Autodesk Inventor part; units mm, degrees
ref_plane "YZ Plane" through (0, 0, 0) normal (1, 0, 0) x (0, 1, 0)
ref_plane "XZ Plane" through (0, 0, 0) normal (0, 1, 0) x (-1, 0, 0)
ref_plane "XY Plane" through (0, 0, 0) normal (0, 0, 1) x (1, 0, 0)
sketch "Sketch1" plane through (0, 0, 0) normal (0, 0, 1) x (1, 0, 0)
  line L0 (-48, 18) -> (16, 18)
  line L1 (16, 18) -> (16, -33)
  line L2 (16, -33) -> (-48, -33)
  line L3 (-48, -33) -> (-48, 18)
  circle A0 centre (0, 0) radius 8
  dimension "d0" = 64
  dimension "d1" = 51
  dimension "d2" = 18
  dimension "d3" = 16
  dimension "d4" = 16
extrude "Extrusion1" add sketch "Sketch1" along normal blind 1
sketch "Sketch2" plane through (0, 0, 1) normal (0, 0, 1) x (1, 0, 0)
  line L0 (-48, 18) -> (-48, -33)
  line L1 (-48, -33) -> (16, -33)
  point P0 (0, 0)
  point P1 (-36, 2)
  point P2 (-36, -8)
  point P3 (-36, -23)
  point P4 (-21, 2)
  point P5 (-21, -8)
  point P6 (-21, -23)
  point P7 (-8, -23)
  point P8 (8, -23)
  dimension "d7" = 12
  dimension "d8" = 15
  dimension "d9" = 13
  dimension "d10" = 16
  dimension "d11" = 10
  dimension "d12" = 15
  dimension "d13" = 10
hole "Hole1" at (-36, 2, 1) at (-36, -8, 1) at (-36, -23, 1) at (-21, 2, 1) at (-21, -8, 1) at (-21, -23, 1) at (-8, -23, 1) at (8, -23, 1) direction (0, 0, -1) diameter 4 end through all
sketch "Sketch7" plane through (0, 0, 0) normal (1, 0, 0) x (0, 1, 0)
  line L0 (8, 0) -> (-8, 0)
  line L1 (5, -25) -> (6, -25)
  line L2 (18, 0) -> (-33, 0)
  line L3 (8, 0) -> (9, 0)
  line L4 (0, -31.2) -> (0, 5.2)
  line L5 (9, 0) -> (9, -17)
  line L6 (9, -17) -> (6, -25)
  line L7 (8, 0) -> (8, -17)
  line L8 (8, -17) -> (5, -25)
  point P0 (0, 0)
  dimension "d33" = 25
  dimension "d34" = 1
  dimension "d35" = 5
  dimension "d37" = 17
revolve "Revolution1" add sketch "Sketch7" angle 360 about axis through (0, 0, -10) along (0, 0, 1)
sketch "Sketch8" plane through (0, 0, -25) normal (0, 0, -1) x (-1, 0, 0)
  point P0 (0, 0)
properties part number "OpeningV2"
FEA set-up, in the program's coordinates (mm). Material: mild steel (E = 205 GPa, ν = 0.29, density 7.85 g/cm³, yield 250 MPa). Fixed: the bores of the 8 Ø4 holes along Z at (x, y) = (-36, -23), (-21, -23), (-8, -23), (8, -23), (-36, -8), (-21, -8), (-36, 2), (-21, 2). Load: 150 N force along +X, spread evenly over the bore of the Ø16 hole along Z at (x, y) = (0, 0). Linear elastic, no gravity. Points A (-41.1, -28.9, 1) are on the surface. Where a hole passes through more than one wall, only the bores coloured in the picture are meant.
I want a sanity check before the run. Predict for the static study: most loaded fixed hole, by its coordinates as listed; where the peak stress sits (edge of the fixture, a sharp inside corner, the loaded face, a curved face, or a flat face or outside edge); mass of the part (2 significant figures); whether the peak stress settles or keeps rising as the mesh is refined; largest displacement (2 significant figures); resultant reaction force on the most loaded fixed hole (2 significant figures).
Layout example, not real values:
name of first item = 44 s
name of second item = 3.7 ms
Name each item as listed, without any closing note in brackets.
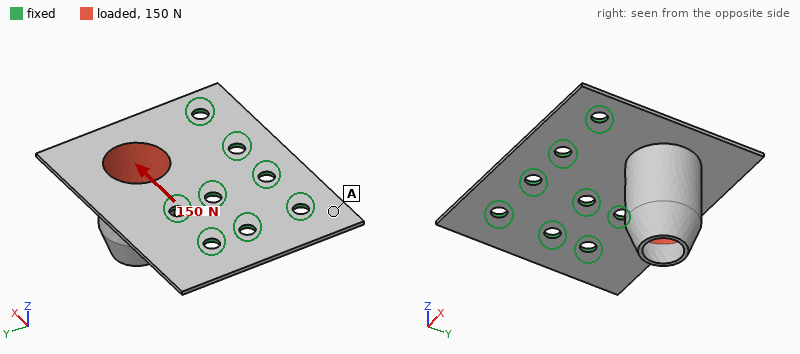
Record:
most loaded fixed hole, by its coordinates as listed = (-21, 2)
where the peak stress sits = edge of the fixture
mass of the part = 33 g
whether the peak stress settles or keeps rising as the mesh is refined = keeps rising
largest displacement = 0.24 mm
resultant reaction force on the most loaded fixed hole = 73 N
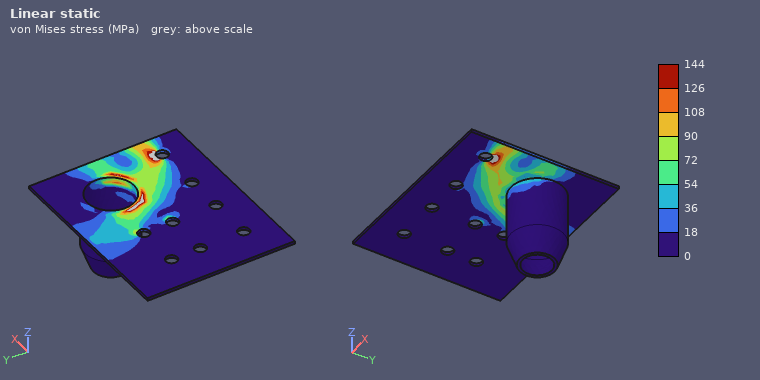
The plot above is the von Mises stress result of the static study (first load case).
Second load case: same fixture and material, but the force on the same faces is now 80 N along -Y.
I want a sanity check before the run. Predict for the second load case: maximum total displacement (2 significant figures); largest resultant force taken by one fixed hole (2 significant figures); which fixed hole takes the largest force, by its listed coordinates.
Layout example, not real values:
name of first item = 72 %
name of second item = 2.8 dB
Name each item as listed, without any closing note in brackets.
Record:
maximum total displacement = 0.13 mm
largest resultant force taken by one fixed hole = 44 N
which fixed hole takes the largest force, by its listed coordinates = (8, -23)
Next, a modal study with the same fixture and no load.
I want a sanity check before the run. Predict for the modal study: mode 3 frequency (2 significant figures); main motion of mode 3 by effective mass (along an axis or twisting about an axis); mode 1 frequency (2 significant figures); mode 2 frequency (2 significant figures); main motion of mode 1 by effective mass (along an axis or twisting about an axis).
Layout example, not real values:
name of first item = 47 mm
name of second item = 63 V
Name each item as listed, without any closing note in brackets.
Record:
mode 3 frequency = 3300 Hz
main motion of mode 3 by effective mass = along Z
mode 1 frequency = 820 Hz
mode 2 frequency = 2100 Hz
main motion of mode 1 by effective mass = along Z
